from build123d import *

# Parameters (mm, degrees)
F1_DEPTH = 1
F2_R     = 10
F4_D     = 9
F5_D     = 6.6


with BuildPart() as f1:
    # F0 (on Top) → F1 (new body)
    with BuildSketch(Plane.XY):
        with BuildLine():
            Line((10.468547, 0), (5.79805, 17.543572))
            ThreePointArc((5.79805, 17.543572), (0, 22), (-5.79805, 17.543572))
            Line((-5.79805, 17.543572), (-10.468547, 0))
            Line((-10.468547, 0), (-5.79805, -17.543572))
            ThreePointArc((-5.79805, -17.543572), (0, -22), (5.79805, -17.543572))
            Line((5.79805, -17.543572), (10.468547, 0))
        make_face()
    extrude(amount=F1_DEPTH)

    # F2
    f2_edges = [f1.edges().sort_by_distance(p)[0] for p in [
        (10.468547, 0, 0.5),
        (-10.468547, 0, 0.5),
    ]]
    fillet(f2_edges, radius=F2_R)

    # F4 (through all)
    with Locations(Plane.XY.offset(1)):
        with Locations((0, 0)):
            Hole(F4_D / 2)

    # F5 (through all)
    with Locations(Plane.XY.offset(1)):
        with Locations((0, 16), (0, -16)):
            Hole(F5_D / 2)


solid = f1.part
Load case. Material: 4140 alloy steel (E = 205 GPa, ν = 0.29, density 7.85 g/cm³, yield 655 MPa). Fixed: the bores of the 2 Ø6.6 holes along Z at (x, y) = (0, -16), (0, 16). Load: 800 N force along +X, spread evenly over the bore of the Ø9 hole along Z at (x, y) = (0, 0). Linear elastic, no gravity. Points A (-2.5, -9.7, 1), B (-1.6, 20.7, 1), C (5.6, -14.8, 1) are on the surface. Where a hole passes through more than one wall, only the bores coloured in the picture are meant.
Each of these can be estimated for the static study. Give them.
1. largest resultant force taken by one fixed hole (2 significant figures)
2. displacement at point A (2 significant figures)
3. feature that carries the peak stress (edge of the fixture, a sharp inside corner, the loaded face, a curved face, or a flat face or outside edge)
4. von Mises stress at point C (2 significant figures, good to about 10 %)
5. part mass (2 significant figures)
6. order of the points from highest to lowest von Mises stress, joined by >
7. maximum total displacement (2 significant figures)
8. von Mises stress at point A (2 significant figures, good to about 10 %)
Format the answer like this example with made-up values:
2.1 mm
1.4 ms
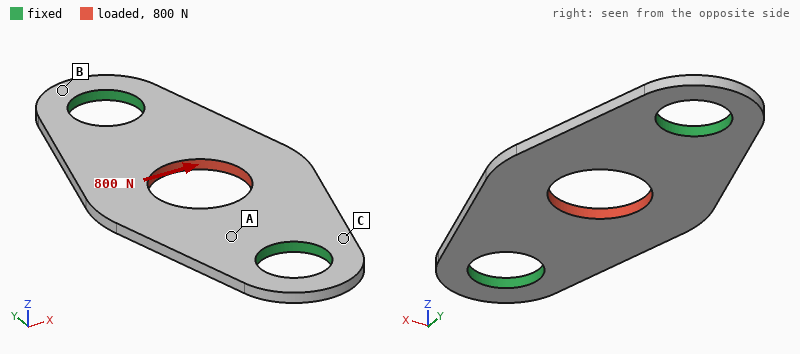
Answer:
400 N
2.2 µm
edge of the fixture
24 MPa
4.0 g
A > C > B
5.9 µm
57 MPa
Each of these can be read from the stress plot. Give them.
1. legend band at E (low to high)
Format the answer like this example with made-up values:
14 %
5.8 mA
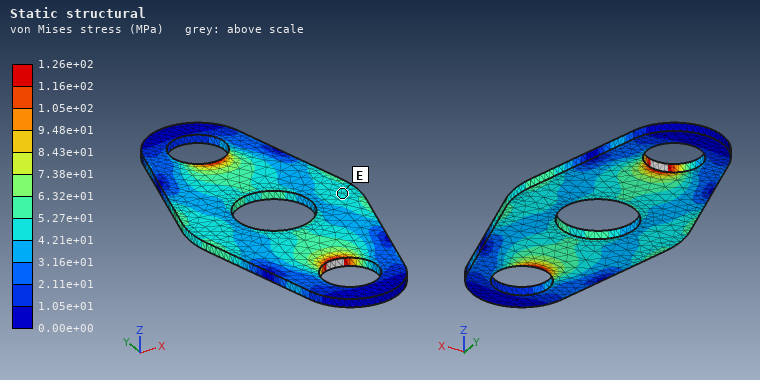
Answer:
4.21e+01 to 5.27e+01 MPa
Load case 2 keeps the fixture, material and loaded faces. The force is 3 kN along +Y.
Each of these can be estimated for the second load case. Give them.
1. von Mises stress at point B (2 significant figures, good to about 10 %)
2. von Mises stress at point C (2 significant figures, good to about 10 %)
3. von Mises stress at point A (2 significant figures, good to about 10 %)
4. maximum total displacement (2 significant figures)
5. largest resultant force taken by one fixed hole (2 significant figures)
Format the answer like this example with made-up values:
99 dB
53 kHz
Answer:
16 MPa
66 MPa
130 MPa
7.9 µm
1.5 kN
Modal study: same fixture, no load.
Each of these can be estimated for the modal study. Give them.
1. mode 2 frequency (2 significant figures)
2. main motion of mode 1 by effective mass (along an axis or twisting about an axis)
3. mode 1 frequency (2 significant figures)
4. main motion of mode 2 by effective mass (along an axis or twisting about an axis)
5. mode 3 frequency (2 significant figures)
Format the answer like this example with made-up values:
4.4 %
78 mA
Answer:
6700 Hz
along Z
6400 Hz
twisting about Y
16 kHz
